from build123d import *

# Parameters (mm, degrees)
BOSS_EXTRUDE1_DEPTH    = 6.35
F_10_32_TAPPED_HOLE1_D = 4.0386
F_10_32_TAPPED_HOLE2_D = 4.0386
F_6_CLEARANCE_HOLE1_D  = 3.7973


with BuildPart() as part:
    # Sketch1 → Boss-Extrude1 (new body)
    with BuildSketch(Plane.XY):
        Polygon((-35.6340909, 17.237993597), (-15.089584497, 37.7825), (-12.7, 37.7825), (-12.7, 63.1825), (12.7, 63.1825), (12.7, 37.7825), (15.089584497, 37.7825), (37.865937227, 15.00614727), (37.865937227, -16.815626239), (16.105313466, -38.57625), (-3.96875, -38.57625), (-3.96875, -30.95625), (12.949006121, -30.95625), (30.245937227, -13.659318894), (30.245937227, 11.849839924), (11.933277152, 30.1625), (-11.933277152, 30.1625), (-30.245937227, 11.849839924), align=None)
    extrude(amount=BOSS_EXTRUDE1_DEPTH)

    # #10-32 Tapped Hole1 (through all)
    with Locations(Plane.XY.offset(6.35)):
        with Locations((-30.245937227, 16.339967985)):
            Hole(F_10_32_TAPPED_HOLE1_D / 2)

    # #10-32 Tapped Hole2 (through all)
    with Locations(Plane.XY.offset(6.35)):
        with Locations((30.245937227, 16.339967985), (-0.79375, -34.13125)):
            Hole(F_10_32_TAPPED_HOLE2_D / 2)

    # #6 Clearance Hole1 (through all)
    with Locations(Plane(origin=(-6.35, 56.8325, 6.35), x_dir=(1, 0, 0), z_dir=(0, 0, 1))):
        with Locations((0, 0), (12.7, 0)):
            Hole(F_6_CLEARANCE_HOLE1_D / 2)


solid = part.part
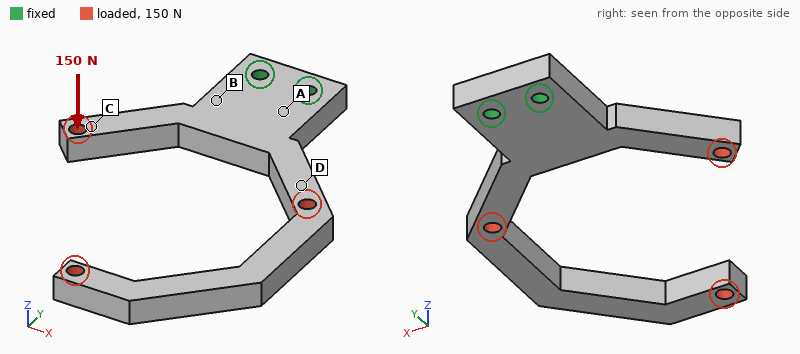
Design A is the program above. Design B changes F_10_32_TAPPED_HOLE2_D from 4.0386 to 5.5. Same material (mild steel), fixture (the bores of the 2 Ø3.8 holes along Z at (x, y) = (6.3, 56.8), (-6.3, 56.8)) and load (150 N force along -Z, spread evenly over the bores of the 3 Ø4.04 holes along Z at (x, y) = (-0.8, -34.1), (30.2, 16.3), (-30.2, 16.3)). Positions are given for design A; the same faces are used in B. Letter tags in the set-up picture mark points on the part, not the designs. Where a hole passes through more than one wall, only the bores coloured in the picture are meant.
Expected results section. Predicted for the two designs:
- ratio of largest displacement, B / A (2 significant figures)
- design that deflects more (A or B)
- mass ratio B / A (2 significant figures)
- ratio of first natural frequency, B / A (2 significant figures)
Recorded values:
1.2
B
0.99
0.96
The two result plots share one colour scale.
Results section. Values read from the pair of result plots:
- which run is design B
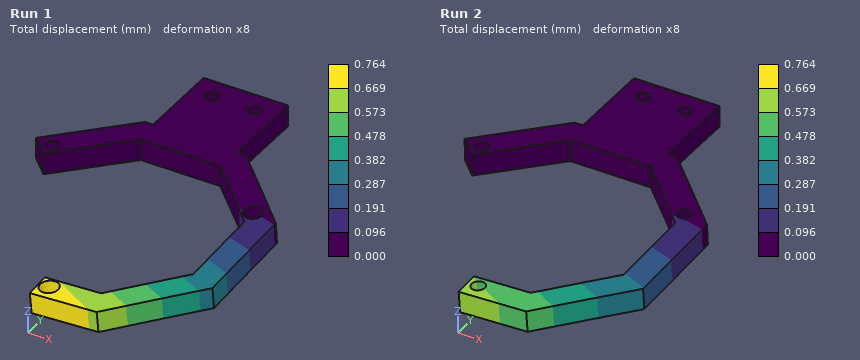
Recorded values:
Run 1
